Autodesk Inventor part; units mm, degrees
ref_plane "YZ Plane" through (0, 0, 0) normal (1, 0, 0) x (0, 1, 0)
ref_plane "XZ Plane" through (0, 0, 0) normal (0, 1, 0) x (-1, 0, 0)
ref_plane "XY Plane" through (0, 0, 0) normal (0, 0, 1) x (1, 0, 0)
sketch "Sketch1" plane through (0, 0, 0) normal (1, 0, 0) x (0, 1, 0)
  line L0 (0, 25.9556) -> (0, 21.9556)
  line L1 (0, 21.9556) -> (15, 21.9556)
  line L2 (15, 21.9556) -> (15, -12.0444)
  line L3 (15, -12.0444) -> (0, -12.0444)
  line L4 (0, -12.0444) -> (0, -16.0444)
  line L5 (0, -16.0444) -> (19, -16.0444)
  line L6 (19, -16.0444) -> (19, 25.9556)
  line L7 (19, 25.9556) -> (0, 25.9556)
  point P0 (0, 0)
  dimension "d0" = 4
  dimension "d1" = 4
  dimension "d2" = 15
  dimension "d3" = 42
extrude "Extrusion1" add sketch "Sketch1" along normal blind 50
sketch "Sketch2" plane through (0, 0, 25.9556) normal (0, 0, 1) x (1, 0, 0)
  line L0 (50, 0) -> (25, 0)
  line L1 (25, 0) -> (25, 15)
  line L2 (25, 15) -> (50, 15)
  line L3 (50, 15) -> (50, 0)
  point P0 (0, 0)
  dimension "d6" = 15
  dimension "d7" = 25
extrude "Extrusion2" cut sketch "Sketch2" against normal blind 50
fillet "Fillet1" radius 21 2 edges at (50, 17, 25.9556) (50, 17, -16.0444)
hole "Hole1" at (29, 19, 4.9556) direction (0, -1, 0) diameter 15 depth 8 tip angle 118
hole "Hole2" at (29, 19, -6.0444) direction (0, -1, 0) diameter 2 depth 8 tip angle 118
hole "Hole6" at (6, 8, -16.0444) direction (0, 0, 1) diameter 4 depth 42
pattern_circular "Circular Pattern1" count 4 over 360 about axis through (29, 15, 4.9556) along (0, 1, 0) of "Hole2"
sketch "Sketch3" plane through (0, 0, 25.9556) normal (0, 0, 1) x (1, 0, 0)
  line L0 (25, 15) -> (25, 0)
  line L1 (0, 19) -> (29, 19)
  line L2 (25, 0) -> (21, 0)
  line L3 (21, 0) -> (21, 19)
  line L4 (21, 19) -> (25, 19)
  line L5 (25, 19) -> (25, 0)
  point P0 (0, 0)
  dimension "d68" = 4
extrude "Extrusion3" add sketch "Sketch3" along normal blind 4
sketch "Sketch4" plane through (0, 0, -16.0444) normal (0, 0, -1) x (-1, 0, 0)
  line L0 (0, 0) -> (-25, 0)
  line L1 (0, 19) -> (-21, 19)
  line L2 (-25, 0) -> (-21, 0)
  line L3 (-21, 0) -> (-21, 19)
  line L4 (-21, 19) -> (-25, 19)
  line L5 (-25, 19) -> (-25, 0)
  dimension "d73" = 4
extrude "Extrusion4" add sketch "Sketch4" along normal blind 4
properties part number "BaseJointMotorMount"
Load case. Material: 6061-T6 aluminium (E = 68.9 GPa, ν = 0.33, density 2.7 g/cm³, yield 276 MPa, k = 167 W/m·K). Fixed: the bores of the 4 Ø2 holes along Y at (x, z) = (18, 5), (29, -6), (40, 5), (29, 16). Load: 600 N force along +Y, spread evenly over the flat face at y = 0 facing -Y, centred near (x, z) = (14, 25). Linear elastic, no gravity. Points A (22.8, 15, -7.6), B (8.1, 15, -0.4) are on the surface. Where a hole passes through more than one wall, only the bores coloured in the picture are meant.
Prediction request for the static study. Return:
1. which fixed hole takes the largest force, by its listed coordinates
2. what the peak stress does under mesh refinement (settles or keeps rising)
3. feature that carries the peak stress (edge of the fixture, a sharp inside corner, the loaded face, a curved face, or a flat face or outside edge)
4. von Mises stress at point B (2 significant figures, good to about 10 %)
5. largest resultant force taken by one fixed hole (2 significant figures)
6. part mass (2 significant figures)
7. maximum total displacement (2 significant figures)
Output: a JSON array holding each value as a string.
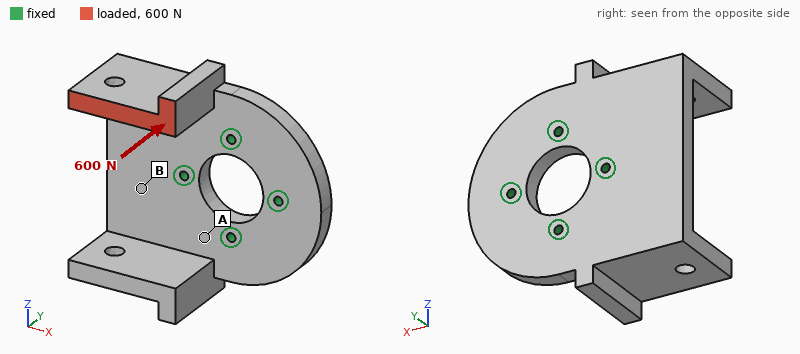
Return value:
["(29, 16)", "keeps rising", "edge of the fixture", "41 MPa", "480 N", "28 g", "0.23 mm"]
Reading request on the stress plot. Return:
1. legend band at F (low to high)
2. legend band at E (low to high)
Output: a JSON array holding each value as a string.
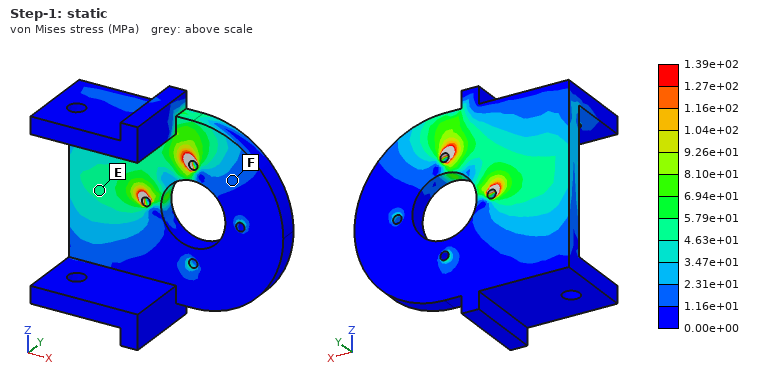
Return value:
["1.16e+01 to 2.31e+01 MPa", "4.63e+01 to 5.79e+01 MPa"]
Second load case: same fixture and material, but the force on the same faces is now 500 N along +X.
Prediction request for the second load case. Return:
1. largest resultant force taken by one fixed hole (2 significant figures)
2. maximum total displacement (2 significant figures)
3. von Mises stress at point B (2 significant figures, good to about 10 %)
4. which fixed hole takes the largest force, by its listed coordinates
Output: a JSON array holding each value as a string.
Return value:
["550 N", "0.21 mm", "39 MPa", "(29, 16)"]
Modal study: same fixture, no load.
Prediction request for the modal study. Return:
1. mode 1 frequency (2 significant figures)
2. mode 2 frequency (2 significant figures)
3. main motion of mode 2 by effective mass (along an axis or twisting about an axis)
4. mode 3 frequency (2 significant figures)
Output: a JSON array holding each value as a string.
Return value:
["3500 Hz", "3800 Hz", "along Y", "6700 Hz"]
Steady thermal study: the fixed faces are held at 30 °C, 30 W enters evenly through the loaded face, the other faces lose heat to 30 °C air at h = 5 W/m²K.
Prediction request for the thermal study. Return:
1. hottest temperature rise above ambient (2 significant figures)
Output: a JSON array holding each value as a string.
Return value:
["52 K"]
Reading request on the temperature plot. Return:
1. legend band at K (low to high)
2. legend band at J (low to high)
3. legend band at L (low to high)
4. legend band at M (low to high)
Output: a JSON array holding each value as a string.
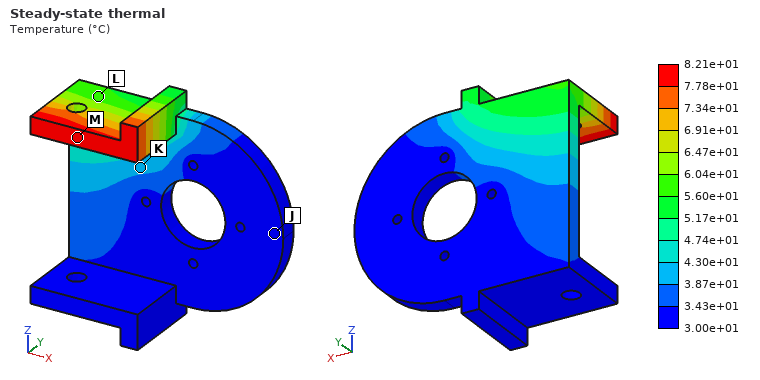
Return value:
["3.87e+01 to 4.30e+01 °C", "3.00e+01 to 3.43e+01 °C", "5.60e+01 to 6.04e+01 °C", "7.78e+01 to 8.21e+01 °C"]
